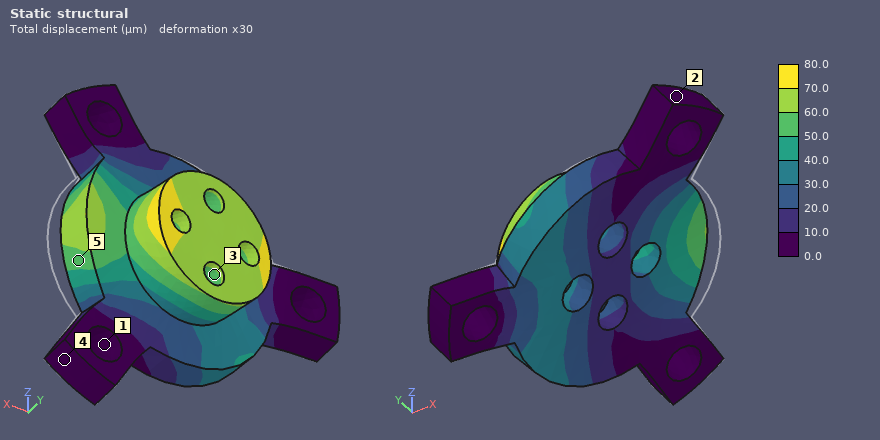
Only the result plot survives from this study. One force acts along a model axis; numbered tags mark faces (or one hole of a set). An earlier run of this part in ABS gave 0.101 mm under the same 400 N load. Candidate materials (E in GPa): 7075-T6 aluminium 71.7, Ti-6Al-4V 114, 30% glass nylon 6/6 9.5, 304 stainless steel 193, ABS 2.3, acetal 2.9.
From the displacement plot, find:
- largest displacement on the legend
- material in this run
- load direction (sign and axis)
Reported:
80.0 µm
acetal
-X
